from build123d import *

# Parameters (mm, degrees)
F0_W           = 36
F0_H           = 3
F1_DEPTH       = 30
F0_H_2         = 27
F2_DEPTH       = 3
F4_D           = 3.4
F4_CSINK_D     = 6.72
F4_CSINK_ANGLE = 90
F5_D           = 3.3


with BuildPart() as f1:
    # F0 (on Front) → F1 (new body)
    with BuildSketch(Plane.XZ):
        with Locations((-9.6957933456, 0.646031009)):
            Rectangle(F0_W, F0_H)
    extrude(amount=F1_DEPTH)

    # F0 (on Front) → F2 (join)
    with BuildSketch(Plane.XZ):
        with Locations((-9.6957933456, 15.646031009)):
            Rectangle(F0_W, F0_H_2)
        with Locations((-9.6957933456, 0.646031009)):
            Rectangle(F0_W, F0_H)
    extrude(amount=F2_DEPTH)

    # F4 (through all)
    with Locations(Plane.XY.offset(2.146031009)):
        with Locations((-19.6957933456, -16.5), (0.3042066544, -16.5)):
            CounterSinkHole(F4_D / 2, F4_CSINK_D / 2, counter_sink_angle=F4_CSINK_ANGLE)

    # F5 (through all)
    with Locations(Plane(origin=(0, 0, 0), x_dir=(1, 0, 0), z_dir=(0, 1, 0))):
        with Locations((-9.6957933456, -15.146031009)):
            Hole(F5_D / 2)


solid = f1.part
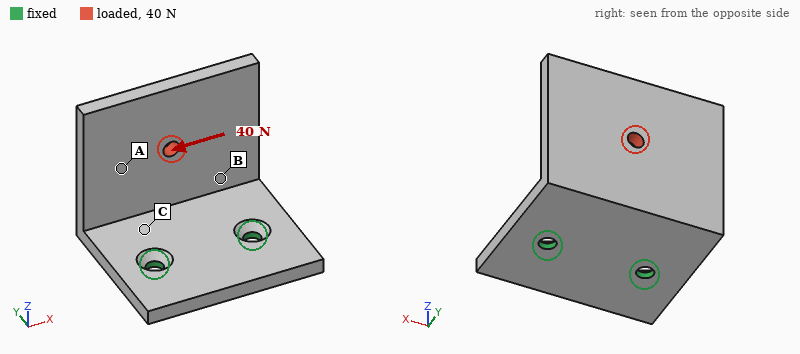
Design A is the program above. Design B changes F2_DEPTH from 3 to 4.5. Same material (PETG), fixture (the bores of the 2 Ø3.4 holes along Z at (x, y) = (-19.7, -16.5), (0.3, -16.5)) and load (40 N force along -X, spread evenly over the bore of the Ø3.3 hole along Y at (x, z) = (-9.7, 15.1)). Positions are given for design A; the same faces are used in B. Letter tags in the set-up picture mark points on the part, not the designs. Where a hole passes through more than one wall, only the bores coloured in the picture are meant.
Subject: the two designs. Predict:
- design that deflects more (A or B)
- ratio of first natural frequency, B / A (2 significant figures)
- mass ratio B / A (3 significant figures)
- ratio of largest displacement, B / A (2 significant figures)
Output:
A
0.90
1.24
0.68
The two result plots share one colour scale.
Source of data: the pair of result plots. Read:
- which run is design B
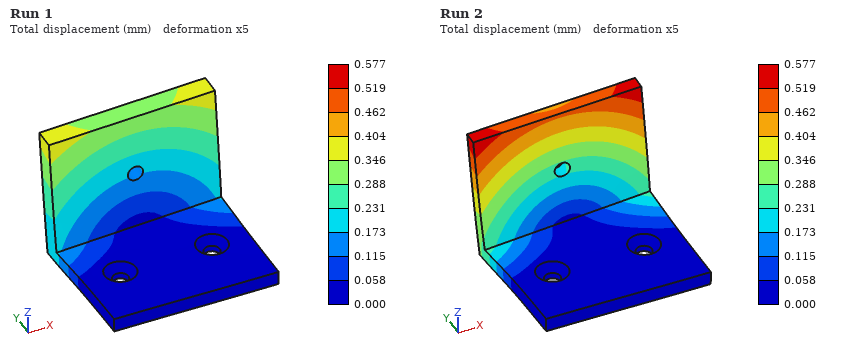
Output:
Run 1
